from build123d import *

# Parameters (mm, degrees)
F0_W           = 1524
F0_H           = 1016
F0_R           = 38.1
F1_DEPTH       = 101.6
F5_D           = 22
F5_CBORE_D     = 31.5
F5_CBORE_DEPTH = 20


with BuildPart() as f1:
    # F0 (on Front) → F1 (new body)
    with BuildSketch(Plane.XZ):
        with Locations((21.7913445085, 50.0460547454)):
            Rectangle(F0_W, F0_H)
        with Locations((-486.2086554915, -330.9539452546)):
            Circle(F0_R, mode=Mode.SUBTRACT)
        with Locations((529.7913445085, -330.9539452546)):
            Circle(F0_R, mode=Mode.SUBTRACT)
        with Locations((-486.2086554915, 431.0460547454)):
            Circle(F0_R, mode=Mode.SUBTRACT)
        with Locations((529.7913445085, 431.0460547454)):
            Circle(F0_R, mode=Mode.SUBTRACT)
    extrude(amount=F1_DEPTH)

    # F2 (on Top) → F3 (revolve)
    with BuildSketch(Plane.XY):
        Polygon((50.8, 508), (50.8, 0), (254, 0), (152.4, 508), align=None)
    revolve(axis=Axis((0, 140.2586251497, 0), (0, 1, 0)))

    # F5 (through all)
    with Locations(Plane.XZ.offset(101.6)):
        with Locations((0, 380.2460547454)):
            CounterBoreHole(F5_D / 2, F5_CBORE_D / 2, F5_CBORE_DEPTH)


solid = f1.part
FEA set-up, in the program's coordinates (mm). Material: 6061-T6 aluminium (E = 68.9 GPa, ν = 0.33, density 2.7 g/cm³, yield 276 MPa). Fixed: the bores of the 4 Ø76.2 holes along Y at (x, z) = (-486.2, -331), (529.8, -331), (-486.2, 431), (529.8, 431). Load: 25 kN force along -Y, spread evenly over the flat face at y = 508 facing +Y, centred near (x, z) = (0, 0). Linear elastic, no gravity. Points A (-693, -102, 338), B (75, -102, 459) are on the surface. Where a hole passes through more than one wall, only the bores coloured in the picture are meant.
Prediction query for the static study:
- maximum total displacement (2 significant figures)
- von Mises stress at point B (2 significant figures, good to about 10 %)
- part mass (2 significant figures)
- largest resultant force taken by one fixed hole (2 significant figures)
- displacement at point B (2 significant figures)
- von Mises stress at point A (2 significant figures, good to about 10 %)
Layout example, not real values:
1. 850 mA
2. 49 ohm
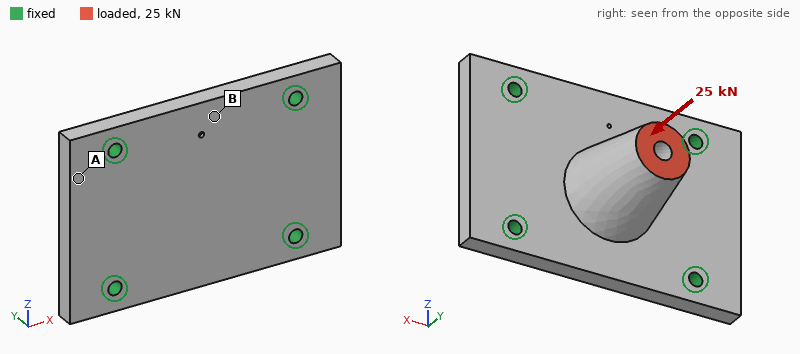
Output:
1. 21 µm
2. 0.65 MPa
3. 590 kg
4. 7.7 kN
5. 13 µm
6. 0.21 MPa
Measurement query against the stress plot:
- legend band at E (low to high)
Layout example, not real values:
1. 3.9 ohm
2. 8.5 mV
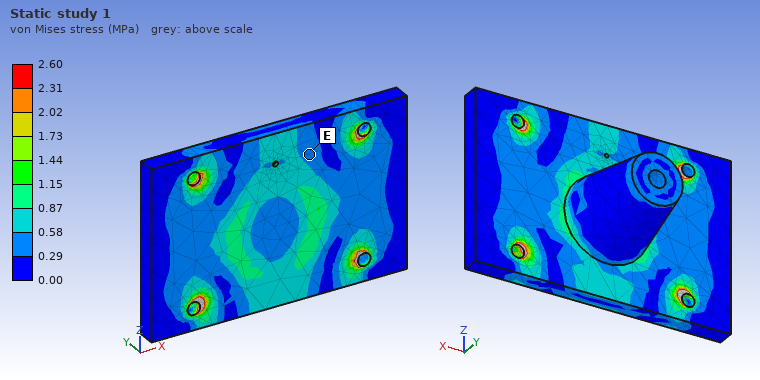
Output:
1. 0.29 to 0.58 MPa
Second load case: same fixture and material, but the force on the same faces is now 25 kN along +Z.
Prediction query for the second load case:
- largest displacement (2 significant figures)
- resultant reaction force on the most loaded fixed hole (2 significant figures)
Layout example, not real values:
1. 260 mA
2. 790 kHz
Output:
1. 79 µm
2. 14 kN
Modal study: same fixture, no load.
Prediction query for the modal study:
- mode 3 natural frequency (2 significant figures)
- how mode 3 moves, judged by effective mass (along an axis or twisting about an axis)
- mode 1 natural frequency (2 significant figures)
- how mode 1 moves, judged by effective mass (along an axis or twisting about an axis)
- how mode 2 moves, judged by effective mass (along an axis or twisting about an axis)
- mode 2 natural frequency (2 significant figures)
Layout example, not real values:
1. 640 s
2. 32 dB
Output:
1. 440 Hz
2. along X
3. 320 Hz
4. along Y
5. along Z
6. 350 Hz
